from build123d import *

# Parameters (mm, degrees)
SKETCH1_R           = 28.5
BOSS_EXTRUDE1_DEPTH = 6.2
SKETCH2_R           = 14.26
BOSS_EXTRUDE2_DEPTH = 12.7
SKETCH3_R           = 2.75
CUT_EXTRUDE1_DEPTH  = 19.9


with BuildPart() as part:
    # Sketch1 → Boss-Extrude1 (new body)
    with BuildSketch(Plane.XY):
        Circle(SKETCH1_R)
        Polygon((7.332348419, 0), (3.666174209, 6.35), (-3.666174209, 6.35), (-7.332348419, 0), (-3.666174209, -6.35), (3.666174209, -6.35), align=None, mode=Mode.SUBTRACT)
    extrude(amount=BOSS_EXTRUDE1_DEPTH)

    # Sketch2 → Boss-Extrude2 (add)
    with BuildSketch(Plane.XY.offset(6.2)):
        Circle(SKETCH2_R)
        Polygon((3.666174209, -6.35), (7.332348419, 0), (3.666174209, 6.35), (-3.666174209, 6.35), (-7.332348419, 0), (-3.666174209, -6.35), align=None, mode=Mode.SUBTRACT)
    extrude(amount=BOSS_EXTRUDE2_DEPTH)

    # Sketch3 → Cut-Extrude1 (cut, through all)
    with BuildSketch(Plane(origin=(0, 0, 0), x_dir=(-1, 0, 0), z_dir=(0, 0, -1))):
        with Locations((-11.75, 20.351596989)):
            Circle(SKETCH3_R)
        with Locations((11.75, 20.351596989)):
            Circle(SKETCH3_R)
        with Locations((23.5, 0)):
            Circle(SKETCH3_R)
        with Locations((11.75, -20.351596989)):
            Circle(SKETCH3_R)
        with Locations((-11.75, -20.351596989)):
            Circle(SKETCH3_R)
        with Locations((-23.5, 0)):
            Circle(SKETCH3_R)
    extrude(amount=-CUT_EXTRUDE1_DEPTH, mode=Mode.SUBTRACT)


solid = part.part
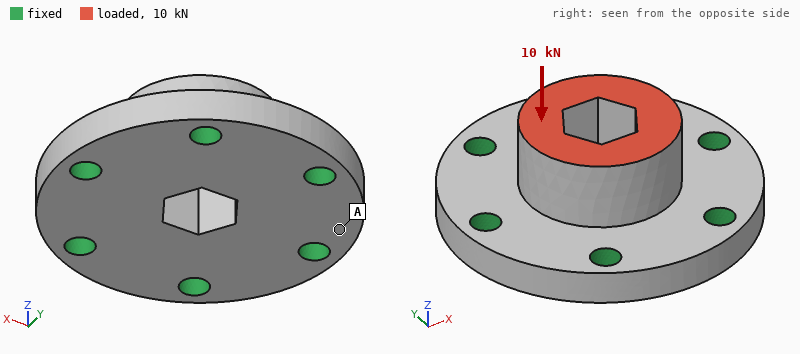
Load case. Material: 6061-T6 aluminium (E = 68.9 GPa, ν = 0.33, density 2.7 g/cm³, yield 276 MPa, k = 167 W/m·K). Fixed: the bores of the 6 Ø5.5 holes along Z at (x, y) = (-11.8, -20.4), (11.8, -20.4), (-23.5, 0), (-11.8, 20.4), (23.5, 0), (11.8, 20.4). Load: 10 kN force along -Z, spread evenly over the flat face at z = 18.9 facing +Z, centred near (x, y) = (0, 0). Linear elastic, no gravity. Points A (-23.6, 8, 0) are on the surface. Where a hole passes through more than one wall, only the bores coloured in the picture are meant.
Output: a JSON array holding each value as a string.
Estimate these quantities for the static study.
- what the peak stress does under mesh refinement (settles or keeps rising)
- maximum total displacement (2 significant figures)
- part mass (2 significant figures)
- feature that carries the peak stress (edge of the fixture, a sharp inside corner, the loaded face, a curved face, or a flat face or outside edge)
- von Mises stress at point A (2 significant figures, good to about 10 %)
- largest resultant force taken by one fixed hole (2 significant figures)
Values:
["keeps rising", "21 µm", "55 g", "edge of the fixture", "18 MPa", "1.8 kN"]
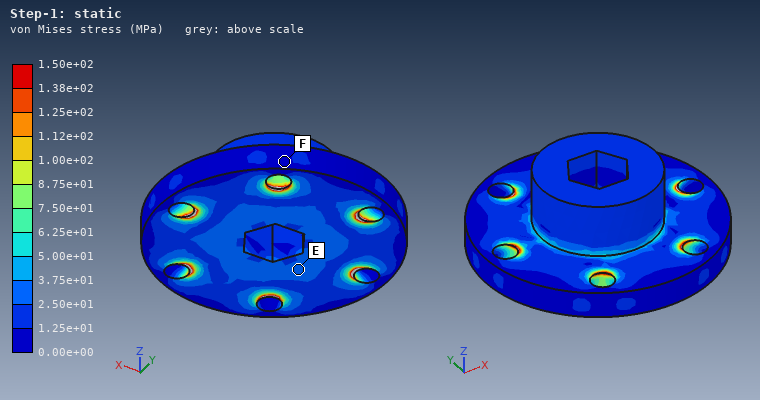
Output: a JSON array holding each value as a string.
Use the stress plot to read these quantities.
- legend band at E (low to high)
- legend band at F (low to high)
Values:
["2.50e+01 to 3.75e+01 MPa", "0.00e+00 to 1.25e+01 MPa"]
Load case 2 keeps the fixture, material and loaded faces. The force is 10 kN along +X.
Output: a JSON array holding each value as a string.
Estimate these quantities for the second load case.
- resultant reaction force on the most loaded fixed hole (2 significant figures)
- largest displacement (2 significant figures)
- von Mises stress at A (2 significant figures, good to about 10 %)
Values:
["3.7 kN", "55 µm", "25 MPa"]
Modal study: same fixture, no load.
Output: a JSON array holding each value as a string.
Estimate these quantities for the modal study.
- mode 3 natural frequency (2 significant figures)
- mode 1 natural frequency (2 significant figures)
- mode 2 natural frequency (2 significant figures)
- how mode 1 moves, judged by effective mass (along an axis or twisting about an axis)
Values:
["24 kHz", "22 kHz", "24 kHz", "along Z"]
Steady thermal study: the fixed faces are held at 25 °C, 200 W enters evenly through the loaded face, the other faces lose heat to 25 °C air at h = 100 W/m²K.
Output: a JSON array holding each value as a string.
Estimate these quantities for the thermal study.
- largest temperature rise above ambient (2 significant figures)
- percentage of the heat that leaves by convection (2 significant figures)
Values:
["54 K", "5.2 %"]
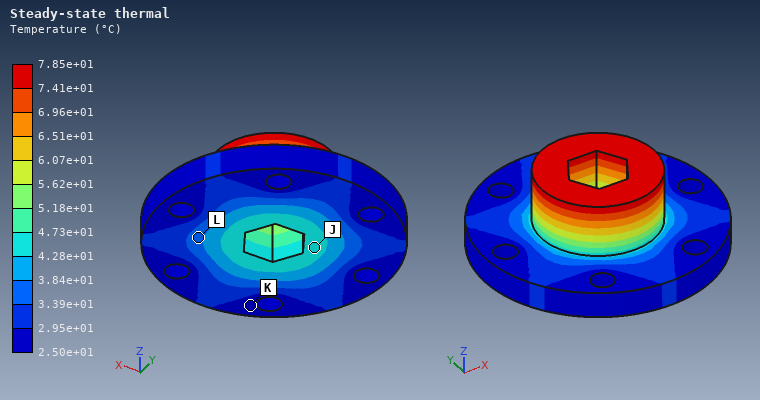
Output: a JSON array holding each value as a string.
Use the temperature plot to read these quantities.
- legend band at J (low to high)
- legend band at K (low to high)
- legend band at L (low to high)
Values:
["4.28e+01 to 4.73e+01 °C", "2.50e+01 to 2.95e+01 °C", "3.39e+01 to 3.84e+01 °C"]
